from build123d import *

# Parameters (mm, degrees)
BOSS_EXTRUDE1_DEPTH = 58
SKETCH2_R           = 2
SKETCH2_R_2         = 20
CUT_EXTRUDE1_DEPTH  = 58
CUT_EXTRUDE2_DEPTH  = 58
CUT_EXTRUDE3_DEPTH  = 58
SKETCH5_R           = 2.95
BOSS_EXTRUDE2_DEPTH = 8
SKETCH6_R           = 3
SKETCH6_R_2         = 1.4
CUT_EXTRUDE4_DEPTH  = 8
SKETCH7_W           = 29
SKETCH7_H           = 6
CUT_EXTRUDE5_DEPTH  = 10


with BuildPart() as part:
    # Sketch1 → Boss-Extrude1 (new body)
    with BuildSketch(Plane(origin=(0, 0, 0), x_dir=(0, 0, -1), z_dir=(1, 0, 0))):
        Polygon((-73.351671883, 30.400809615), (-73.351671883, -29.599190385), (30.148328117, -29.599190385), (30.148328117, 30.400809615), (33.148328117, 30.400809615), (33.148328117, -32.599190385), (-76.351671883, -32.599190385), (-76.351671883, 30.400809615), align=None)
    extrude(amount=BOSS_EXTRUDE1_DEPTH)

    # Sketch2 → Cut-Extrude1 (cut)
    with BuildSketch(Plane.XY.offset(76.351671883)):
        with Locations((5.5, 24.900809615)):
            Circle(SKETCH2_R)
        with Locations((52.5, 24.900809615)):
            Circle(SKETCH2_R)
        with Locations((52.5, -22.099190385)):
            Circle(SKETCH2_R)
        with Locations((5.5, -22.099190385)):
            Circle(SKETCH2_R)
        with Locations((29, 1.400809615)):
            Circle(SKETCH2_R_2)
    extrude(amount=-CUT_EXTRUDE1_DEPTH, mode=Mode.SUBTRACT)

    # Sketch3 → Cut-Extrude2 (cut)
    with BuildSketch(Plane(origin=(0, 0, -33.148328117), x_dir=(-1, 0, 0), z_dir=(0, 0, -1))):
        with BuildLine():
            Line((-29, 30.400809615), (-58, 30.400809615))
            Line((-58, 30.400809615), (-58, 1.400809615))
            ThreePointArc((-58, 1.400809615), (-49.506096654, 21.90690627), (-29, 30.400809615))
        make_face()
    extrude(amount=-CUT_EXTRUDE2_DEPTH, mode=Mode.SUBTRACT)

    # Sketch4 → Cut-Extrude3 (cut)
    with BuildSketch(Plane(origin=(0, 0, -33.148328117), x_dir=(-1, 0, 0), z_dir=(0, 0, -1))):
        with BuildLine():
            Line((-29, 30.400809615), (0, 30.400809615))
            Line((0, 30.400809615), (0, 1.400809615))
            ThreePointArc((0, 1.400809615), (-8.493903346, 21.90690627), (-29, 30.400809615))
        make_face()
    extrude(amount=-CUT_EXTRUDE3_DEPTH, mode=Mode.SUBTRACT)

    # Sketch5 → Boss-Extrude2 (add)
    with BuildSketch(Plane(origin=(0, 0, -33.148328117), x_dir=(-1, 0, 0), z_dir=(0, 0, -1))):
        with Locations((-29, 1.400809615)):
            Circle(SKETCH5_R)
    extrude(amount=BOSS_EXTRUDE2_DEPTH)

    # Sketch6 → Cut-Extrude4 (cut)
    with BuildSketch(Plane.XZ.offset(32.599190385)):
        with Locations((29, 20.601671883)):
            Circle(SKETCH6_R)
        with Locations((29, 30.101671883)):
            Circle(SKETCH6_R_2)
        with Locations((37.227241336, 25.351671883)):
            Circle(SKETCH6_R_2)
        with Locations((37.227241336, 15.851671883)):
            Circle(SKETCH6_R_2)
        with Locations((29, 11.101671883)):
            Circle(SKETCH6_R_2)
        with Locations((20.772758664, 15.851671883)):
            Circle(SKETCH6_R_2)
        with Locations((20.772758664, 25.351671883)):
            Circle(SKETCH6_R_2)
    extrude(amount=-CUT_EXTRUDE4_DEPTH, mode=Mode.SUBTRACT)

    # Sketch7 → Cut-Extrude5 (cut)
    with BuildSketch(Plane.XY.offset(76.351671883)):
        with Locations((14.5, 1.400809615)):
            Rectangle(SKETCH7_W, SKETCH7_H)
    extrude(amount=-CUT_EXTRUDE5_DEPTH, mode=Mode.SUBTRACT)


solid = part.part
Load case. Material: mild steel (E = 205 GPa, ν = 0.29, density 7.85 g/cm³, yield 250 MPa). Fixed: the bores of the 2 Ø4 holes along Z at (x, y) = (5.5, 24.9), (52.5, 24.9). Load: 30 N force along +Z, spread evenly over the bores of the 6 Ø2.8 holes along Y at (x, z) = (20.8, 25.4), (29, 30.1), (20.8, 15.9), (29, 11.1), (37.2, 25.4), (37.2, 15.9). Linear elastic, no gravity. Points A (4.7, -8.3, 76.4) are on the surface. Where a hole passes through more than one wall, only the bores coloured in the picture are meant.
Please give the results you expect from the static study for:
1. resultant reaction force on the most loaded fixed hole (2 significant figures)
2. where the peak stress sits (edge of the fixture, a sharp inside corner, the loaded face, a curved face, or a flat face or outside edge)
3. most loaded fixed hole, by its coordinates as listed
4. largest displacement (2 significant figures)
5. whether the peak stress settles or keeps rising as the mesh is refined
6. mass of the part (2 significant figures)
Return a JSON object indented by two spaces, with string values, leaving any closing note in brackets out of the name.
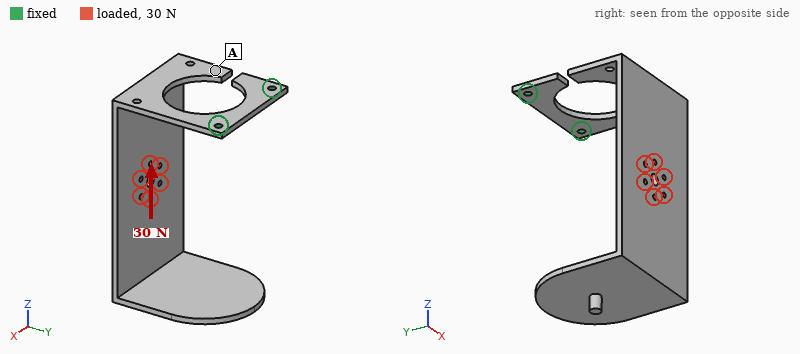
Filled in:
{
  "resultant reaction force on the most loaded fixed hole": "30 N",
  "where the peak stress sits": "edge of the fixture",
  "most loaded fixed hole, by its coordinates as listed": "(52.5, 24.9)",
  "largest displacement": "1.2 mm",
  "whether the peak stress settles or keeps rising as the mesh is refined": "keeps rising",
  "mass of the part": "270 g"
}
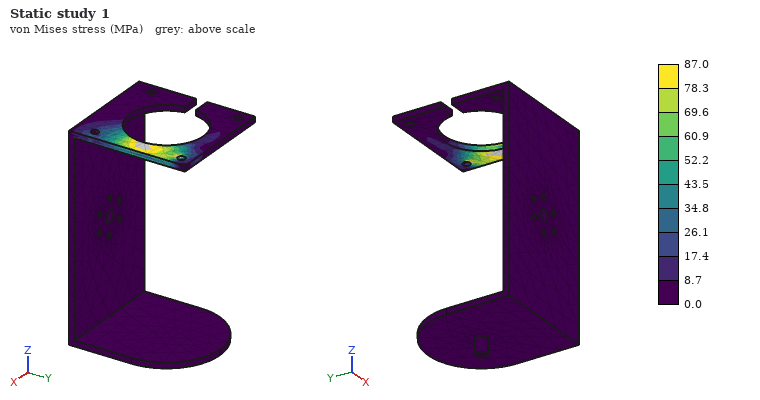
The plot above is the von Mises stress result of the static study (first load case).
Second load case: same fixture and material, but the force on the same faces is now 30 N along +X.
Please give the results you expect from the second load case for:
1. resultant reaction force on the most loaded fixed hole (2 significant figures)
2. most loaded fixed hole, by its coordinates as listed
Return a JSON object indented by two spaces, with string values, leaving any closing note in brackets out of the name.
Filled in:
{
  "resultant reaction force on the most loaded fixed hole": "35 N",
  "most loaded fixed hole, by its coordinates as listed": "(52.5, 24.9)"
}
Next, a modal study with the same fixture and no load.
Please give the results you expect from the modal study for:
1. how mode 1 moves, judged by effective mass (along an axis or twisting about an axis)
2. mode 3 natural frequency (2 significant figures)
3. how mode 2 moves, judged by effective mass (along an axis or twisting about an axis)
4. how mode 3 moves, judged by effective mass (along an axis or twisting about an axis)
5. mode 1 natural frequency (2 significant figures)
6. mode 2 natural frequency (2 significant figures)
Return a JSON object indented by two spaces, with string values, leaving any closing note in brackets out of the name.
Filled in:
{
  "how mode 1 moves, judged by effective mass": "along Y",
  "mode 3 natural frequency": "180 Hz",
  "how mode 2 moves, judged by effective mass": "along X",
  "how mode 3 moves, judged by effective mass": "along Z",
  "mode 1 natural frequency": "39 Hz",
  "mode 2 natural frequency": "48 Hz"
}
